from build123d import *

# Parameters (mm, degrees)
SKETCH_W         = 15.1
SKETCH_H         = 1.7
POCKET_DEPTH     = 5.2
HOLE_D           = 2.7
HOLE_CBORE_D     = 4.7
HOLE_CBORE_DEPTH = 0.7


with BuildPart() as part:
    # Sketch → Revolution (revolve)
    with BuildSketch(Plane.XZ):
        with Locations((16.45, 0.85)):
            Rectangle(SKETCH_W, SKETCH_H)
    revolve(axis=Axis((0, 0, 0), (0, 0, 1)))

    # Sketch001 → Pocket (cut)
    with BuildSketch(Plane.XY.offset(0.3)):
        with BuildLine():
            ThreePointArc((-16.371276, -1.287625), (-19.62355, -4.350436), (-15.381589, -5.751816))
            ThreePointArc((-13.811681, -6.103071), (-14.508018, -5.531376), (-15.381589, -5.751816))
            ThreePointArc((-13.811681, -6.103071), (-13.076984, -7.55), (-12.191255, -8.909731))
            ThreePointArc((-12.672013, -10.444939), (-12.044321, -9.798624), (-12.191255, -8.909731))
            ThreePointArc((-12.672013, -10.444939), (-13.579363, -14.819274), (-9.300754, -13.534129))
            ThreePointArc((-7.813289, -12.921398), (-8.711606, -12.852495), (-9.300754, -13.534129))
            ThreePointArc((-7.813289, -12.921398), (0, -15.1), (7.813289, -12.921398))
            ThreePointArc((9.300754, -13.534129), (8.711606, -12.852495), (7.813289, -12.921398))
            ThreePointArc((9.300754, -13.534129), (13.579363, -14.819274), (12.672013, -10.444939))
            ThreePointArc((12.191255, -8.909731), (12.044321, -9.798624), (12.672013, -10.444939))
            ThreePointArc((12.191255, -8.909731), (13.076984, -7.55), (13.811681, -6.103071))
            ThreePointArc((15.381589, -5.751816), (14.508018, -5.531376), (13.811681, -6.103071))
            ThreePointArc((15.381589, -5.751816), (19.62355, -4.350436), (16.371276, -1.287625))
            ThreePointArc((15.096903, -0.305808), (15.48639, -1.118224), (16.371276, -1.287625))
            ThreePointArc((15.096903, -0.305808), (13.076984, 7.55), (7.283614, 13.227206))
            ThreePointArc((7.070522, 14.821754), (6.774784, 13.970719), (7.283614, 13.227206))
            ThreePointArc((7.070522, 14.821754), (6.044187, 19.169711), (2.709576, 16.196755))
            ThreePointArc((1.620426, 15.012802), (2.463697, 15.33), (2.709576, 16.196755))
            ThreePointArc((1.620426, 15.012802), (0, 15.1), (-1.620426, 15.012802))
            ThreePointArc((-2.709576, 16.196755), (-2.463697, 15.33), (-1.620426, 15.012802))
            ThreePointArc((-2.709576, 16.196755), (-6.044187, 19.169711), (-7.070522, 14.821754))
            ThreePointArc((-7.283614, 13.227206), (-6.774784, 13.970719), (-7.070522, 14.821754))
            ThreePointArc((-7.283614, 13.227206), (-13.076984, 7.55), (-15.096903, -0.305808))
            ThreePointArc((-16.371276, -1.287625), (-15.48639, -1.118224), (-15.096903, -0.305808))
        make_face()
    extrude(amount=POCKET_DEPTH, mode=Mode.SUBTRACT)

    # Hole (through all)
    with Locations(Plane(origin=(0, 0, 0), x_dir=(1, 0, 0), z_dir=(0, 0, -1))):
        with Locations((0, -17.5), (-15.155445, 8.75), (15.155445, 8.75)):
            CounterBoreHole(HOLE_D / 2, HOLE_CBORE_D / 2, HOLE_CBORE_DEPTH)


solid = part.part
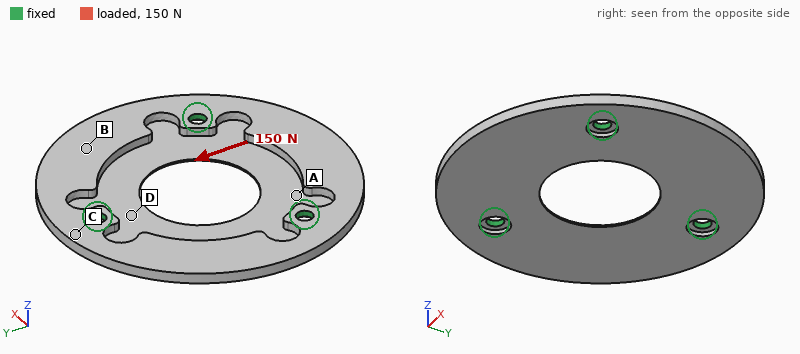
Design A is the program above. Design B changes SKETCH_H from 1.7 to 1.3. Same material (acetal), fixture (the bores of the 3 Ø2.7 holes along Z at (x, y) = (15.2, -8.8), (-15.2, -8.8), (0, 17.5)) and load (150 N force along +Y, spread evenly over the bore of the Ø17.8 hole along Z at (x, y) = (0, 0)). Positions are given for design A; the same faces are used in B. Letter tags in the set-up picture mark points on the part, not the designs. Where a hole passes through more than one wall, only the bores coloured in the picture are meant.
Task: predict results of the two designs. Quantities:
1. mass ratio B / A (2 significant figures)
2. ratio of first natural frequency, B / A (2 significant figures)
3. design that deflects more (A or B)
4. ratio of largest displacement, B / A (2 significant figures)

0.72
0.78
B
2.0
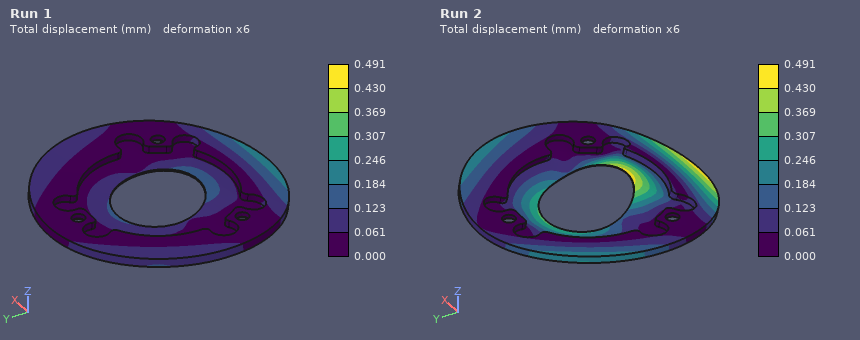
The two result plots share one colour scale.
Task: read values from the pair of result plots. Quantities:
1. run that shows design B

Run 2
